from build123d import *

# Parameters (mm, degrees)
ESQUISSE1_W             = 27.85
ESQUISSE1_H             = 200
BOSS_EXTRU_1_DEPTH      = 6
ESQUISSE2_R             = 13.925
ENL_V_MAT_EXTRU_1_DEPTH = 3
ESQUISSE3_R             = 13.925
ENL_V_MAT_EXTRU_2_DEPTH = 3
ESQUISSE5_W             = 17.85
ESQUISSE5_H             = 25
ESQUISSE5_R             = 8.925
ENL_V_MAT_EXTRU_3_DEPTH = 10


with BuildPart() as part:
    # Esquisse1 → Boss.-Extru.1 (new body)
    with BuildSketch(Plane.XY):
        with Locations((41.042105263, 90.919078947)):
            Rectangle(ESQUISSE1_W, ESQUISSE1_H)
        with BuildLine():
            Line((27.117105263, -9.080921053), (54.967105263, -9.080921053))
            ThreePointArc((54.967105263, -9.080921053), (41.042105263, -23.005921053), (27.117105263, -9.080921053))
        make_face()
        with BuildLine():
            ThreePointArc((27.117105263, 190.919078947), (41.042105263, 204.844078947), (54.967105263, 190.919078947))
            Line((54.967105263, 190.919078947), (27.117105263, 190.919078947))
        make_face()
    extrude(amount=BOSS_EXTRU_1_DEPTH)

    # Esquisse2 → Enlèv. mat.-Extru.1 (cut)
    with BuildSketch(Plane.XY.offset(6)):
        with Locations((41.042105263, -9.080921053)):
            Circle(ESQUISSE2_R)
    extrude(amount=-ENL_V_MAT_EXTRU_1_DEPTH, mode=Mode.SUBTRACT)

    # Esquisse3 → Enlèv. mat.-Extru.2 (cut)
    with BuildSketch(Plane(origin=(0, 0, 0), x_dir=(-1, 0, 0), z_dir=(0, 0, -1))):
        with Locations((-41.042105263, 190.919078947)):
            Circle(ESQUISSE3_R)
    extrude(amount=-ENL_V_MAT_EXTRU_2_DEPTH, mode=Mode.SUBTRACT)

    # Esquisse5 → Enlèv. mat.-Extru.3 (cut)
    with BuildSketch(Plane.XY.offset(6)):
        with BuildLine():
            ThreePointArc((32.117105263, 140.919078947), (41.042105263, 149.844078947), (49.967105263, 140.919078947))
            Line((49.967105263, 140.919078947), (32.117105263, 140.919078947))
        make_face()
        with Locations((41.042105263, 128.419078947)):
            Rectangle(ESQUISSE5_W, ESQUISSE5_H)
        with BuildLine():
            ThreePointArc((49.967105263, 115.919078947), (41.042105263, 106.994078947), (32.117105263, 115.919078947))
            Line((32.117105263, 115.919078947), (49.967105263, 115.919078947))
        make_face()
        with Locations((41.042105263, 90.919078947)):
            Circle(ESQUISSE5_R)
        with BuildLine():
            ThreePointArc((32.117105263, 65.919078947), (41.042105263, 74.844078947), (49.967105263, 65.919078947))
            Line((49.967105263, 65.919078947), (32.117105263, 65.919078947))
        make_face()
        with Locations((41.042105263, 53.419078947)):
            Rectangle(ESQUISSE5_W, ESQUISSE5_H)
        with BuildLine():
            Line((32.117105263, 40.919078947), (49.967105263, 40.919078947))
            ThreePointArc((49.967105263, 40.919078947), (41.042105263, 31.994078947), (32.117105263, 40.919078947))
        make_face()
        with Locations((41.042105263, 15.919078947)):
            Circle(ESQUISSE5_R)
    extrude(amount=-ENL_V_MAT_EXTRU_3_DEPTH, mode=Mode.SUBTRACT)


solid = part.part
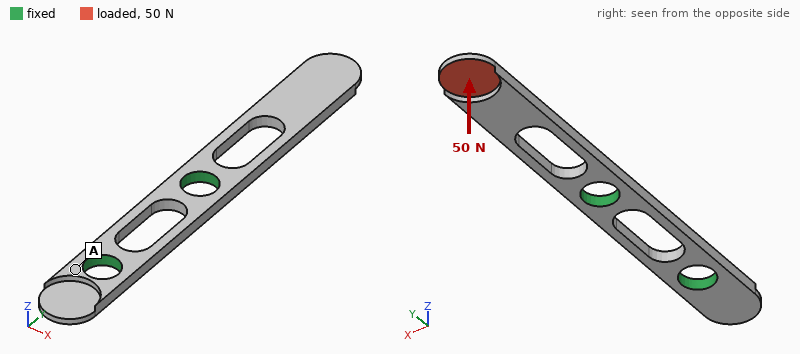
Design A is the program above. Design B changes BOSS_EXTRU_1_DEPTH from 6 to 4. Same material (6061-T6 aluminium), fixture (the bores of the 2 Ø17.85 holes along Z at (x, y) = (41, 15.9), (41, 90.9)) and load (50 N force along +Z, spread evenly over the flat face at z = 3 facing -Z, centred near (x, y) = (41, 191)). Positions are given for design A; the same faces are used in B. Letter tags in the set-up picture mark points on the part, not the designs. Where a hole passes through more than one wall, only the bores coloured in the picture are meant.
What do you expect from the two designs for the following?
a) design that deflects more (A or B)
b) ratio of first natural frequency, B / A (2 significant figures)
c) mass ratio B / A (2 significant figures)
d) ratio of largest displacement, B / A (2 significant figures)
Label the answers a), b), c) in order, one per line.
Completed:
a) B
b) 0.77
c) 0.67
d) 3.6
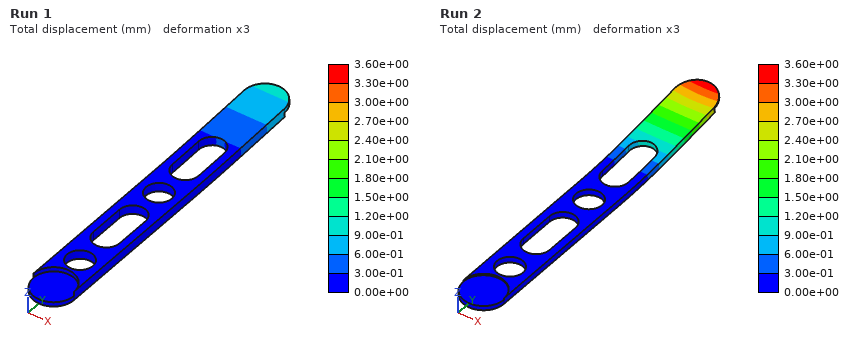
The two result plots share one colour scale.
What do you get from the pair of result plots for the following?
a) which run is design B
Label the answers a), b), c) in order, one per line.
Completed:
a) Run 2
